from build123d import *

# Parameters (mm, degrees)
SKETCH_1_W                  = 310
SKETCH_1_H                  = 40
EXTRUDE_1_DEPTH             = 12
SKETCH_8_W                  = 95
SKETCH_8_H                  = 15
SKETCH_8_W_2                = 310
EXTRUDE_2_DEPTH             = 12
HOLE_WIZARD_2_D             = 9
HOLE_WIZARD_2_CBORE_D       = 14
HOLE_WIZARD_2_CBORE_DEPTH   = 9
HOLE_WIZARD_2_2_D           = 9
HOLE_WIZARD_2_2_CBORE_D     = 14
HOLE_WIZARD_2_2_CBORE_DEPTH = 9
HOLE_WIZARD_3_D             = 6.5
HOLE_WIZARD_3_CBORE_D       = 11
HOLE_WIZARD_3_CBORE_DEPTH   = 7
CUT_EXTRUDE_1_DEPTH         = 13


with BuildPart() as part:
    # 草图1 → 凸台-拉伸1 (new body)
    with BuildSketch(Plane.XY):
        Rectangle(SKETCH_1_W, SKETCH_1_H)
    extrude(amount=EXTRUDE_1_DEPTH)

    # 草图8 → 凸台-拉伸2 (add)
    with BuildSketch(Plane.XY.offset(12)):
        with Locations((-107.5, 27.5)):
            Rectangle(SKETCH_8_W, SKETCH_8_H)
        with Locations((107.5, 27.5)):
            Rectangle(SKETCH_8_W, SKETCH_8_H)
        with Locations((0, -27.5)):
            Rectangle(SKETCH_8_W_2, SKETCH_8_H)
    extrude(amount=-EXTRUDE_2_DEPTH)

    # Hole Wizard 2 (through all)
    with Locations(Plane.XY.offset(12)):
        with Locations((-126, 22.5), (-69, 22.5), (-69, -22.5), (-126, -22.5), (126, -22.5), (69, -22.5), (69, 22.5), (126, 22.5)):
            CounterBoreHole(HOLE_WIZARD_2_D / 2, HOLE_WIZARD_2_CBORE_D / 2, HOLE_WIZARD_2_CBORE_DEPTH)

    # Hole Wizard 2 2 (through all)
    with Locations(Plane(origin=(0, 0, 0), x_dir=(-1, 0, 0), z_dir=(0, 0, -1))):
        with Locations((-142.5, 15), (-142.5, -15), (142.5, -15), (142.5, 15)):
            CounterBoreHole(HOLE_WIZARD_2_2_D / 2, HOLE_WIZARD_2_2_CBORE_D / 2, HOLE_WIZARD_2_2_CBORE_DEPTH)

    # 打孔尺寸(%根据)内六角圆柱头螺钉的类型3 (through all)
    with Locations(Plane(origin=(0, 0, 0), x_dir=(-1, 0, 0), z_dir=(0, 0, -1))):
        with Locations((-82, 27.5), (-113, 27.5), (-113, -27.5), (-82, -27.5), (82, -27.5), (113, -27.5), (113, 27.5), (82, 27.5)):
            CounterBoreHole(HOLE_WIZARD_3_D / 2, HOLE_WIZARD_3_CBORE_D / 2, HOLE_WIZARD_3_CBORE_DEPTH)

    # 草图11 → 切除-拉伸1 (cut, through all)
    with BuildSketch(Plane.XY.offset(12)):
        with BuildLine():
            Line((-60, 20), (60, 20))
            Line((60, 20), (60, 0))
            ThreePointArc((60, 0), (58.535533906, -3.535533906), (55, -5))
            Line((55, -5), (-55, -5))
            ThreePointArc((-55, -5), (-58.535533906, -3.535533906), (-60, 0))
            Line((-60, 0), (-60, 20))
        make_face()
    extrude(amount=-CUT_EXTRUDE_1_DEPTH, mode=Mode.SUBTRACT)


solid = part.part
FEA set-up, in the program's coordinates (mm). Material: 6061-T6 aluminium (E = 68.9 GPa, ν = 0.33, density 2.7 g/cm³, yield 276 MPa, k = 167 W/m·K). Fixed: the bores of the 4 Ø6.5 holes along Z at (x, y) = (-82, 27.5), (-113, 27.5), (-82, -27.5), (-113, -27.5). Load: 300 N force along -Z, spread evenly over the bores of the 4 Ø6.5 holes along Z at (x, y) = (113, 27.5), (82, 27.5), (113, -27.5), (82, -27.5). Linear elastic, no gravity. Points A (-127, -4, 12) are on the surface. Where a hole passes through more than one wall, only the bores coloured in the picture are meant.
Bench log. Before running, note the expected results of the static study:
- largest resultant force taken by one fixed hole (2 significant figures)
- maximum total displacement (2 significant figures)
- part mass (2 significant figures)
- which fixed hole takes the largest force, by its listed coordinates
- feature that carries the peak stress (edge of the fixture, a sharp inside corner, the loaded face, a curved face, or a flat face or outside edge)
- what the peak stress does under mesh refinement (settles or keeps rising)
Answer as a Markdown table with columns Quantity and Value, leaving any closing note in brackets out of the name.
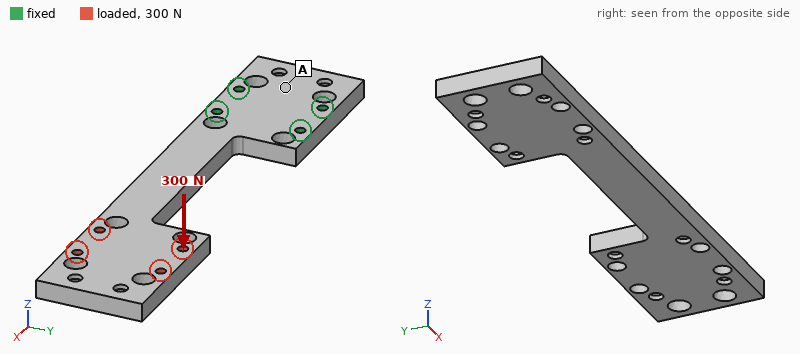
| Quantity | Value |
|---|---|
| largest resultant force taken by one fixed hole | 1.4 kN |
| maximum total displacement | 3.4 mm |
| part mass | 480 g |
| which fixed hole takes the largest force, by its listed coordinates | (-82, -27.5) |
| feature that carries the peak stress | edge of the fixture |
| what the peak stress does under mesh refinement | keeps rising |
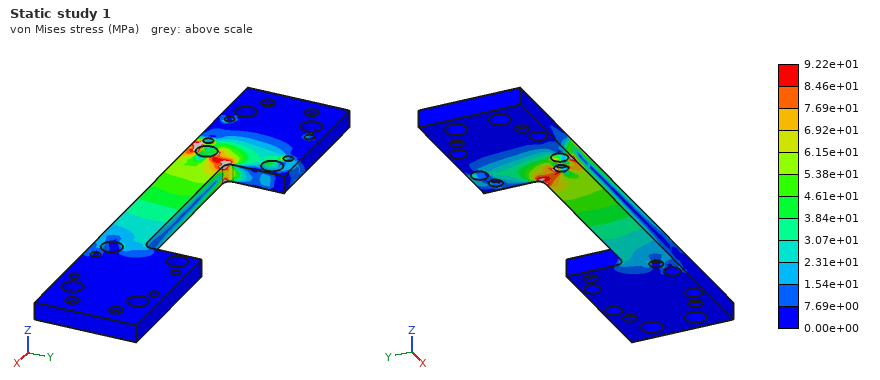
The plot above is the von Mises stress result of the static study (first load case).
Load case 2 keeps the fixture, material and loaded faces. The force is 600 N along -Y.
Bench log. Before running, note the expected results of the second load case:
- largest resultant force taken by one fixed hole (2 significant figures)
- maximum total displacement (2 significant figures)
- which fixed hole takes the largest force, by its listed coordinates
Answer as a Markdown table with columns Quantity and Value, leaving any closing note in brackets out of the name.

| Quantity | Value |
|---|---|
| largest resultant force taken by one fixed hole | 1.9 kN |
| maximum total displacement | 0.95 mm |
| which fixed hole takes the largest force, by its listed coordinates | (-82, -27.5) |
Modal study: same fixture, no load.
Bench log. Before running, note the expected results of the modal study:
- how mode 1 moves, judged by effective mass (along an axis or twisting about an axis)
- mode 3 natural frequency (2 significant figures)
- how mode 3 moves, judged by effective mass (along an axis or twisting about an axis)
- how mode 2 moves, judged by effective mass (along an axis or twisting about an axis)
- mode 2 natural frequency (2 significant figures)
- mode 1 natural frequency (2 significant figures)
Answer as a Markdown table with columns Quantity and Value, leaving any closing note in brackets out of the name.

| Quantity | Value |
|---|---|
| how mode 1 moves, judged by effective mass | along Z |
| mode 3 natural frequency | 780 Hz |
| how mode 3 moves, judged by effective mass | twisting about X |
| how mode 2 moves, judged by effective mass | along Y |
| mode 2 natural frequency | 320 Hz |
| mode 1 natural frequency | 120 Hz |
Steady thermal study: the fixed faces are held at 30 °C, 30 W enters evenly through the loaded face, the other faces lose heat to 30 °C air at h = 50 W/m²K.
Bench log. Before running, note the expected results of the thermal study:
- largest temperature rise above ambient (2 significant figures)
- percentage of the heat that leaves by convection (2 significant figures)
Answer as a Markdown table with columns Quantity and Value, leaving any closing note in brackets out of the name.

| Quantity | Value |
|---|---|
| largest temperature rise above ambient | 24 K |
| percentage of the heat that leaves by convection | 83 % |
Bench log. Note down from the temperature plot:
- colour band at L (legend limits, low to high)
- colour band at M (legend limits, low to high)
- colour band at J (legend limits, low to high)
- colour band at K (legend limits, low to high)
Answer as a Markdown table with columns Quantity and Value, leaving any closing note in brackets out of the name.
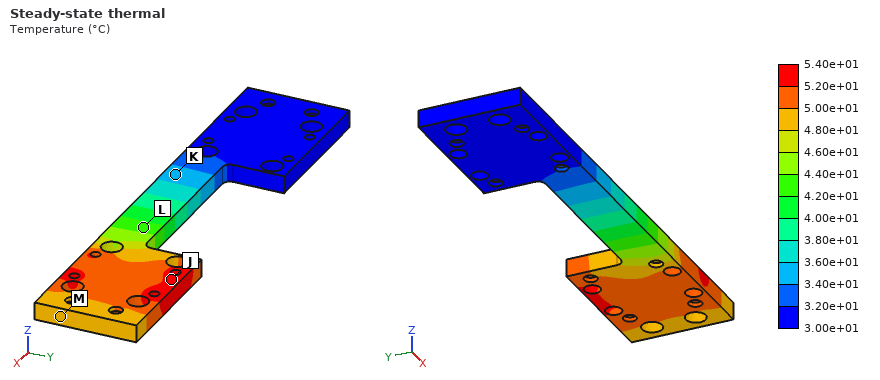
| Quantity | Value |
|---|---|
| colour band at L | 4.20e+01 to 4.40e+01 °C |
| colour band at M | 4.80e+01 to 5.00e+01 °C |
| colour band at J | 5.20e+01 to 5.40e+01 °C |
| colour band at K | 3.40e+01 to 3.60e+01 °C |
